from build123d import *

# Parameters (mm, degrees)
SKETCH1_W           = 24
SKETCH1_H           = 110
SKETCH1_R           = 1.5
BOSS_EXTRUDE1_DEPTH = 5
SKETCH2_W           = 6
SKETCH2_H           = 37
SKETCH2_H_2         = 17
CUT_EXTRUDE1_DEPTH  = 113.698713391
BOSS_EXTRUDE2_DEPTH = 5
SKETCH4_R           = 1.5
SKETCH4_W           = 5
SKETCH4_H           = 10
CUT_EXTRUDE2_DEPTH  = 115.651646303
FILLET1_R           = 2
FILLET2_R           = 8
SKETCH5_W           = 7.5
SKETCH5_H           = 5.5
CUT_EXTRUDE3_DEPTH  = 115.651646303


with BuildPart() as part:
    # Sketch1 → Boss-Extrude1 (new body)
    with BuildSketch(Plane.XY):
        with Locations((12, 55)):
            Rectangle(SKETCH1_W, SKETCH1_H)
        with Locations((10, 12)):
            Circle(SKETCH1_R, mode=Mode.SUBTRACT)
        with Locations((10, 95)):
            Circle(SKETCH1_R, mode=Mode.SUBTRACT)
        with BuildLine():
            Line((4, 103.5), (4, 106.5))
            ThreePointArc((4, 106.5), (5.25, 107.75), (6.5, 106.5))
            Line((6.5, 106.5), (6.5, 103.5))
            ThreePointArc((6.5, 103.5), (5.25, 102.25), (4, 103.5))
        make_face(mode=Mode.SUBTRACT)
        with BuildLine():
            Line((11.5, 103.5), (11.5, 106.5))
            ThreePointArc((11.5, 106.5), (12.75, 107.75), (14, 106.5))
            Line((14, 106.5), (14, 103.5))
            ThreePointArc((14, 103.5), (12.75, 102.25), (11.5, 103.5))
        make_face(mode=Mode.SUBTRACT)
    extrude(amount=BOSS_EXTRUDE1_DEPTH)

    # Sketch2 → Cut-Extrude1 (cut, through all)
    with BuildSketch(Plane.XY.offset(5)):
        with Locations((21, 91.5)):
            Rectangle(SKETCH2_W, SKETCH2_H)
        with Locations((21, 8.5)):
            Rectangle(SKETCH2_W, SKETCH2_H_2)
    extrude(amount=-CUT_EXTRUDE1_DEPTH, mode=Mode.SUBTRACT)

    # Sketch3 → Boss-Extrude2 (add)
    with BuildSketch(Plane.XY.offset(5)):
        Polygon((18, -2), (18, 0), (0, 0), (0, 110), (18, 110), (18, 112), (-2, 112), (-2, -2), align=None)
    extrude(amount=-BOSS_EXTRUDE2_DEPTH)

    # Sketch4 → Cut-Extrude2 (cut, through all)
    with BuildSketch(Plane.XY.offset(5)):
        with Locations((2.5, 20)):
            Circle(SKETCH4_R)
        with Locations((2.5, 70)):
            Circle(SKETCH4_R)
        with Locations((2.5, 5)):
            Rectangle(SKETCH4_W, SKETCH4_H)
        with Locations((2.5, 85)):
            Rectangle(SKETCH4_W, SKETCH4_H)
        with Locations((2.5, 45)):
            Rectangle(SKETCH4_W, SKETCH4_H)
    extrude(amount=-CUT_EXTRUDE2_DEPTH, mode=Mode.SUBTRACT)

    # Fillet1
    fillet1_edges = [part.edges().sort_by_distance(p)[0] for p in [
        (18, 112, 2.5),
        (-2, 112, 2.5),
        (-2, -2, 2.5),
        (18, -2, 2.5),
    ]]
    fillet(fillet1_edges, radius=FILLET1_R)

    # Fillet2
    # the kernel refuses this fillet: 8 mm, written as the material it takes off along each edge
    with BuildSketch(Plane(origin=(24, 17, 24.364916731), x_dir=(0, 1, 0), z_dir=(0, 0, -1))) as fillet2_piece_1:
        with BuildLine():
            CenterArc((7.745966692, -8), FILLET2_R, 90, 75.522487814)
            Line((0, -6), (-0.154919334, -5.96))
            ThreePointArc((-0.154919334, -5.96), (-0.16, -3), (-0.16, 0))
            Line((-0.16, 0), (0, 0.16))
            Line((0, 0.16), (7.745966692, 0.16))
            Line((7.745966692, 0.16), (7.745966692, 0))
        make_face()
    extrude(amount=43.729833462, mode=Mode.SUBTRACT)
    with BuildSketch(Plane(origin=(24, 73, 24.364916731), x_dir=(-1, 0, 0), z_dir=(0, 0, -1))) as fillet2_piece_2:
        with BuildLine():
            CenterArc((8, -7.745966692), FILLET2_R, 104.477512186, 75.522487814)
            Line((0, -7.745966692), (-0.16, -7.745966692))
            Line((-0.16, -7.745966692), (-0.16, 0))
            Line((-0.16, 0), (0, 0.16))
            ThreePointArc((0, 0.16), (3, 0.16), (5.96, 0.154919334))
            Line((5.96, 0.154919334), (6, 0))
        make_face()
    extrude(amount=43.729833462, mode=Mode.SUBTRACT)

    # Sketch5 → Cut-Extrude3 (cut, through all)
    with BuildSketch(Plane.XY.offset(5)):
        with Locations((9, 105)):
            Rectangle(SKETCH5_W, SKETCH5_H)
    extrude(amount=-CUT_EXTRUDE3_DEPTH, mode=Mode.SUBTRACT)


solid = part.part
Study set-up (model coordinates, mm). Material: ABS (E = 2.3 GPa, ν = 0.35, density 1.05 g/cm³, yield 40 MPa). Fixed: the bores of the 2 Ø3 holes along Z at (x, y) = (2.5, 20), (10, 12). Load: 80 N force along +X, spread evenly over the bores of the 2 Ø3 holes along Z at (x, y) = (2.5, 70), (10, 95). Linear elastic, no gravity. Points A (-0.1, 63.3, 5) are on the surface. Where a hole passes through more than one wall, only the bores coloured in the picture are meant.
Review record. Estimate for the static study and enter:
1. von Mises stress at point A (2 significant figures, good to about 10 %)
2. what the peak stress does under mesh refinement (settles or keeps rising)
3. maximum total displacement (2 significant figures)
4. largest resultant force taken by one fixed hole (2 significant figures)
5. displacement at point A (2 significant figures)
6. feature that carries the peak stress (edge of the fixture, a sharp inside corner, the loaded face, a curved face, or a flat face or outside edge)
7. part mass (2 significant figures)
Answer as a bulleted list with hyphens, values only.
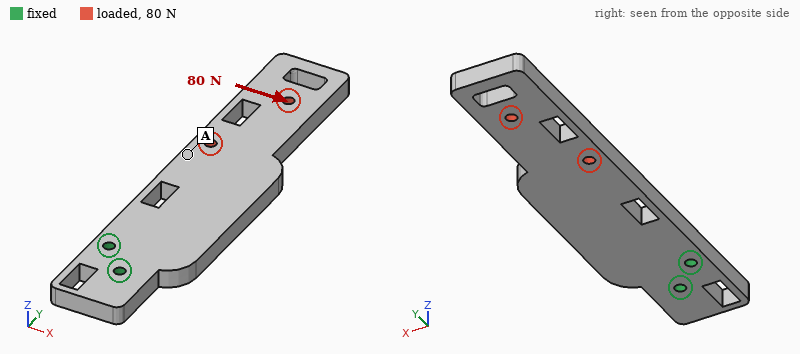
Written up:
- 2.6 MPa
- keeps rising
- 1.4 mm
- 440 N
- 0.53 mm
- edge of the fixture
- 12 g
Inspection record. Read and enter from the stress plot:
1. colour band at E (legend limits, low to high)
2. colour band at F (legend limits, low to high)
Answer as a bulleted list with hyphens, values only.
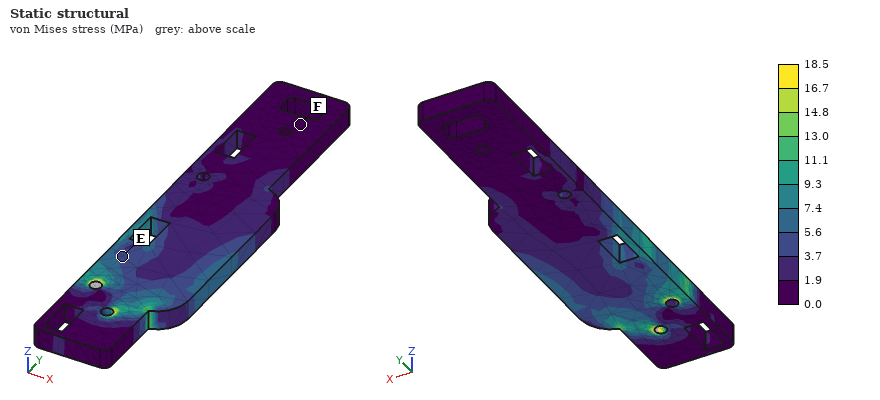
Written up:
- 3.7 to 5.6 MPa
- 0.0 to 1.9 MPa
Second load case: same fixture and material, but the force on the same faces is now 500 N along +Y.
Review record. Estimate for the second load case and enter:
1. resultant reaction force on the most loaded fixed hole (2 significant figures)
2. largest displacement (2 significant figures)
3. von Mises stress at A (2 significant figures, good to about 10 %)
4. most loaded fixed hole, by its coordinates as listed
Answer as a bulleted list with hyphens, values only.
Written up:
- 300 N
- 0.54 mm
- 7.2 MPa
- (2.5, 20)
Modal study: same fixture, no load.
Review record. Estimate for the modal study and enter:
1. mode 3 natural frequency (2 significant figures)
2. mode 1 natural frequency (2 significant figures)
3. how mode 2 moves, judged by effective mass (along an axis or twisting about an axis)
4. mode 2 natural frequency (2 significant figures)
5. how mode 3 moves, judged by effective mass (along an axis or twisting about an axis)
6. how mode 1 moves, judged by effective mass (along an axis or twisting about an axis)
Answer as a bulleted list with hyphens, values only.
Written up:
- 780 Hz
- 160 Hz
- along X
- 600 Hz
- along Z
- along Z
